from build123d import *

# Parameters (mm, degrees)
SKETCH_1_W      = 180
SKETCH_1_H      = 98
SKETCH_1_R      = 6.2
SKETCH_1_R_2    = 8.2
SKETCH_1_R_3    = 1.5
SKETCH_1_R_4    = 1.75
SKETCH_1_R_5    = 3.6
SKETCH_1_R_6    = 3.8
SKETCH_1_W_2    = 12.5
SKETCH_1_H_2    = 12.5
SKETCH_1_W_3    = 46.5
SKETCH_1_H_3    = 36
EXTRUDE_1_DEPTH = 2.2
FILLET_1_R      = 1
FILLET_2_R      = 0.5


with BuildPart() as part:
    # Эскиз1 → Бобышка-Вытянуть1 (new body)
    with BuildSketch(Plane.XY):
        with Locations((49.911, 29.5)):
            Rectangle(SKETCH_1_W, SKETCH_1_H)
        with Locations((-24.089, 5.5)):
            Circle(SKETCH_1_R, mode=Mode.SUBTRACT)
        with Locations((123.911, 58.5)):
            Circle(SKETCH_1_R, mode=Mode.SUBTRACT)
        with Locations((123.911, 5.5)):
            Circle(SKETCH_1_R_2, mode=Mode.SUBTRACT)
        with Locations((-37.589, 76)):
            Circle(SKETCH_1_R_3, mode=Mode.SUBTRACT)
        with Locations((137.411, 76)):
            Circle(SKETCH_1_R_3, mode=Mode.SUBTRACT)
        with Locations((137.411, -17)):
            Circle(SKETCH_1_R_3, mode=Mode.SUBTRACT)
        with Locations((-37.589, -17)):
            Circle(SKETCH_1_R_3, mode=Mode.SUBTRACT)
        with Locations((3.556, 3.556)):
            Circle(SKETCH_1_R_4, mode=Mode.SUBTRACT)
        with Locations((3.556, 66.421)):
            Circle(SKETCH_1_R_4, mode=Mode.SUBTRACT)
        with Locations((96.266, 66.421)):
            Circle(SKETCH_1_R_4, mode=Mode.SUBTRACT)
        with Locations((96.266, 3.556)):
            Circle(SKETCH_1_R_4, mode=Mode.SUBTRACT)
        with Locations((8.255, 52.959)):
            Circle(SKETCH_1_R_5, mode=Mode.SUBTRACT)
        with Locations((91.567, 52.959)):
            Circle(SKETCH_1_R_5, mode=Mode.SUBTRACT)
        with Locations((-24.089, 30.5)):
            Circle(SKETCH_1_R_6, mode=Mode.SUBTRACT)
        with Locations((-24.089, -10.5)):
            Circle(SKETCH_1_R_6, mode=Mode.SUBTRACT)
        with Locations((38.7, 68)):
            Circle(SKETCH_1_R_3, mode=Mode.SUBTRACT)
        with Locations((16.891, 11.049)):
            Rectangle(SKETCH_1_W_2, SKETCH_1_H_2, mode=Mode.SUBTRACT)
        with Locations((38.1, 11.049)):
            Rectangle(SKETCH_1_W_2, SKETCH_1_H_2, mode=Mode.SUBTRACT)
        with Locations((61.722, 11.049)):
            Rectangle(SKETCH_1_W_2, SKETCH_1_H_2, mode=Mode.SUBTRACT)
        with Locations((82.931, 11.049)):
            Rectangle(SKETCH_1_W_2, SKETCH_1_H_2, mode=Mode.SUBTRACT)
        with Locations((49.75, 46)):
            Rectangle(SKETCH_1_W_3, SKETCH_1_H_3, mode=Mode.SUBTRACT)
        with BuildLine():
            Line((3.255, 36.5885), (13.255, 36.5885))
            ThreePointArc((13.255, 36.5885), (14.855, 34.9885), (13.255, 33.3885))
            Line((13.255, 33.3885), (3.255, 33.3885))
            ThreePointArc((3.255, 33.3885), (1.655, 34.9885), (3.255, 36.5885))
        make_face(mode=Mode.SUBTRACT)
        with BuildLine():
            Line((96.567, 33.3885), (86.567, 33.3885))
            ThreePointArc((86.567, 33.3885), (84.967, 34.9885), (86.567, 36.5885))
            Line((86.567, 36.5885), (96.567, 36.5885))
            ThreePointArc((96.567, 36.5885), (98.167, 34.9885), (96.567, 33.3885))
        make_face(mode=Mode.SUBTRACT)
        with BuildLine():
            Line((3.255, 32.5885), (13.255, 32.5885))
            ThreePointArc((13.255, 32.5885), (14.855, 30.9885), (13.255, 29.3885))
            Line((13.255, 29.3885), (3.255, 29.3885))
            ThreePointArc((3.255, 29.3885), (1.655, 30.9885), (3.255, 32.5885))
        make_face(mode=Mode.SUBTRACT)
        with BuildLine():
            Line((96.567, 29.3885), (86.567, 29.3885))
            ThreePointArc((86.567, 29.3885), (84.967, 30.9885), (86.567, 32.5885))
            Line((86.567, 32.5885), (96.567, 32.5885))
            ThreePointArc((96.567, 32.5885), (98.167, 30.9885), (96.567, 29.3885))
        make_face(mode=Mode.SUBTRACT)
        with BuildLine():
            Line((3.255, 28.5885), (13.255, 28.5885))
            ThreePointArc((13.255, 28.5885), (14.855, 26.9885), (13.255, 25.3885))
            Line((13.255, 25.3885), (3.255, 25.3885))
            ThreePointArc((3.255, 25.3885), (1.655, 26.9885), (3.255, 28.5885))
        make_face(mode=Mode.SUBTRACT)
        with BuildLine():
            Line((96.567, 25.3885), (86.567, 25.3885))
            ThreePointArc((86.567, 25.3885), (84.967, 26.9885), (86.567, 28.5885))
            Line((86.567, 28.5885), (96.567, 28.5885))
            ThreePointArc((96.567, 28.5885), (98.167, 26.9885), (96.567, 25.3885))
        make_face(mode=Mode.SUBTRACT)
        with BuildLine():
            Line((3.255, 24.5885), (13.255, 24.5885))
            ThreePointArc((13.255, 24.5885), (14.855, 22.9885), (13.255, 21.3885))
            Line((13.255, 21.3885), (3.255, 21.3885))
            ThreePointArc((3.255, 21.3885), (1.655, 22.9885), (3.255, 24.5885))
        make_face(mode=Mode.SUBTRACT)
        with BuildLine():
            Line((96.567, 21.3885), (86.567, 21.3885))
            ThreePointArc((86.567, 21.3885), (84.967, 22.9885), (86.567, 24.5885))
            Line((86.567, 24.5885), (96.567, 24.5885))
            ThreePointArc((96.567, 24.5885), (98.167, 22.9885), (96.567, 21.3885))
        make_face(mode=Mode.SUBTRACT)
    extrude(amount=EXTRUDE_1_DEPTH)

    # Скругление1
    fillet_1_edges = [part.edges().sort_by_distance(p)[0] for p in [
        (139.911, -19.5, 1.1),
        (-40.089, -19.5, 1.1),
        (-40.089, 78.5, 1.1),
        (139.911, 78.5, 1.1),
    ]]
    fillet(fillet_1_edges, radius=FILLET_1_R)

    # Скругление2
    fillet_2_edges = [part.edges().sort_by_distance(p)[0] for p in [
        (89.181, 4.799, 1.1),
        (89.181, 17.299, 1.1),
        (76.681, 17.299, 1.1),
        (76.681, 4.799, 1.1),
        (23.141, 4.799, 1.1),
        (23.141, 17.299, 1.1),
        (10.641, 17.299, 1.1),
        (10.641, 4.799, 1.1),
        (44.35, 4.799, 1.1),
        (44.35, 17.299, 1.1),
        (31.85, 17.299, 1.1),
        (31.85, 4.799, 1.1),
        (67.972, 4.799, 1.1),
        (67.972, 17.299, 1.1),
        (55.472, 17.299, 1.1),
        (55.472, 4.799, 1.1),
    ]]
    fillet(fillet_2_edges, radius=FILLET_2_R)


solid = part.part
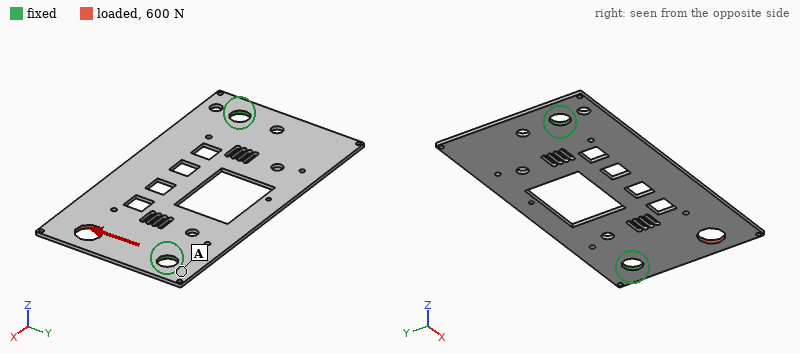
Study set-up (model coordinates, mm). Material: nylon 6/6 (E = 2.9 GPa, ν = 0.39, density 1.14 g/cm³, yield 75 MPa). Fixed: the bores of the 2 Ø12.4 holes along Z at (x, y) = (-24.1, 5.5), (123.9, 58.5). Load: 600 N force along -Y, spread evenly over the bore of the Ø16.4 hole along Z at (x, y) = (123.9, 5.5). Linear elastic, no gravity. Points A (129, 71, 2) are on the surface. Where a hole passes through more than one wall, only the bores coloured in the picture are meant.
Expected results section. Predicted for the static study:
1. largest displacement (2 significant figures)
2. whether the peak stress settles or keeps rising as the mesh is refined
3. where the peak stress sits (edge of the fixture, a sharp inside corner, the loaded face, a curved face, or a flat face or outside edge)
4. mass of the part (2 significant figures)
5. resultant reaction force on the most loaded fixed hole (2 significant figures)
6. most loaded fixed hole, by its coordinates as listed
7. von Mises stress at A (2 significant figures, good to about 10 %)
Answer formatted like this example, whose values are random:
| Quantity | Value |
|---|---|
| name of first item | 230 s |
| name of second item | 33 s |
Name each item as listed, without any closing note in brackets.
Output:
| Quantity | Value |
|---|---|
| largest displacement | 0.20 mm |
| whether the peak stress settles or keeps rising as the mesh is refined | keeps rising |
| where the peak stress sits | a sharp inside corner |
| mass of the part | 36 g |
| resultant reaction force on the most loaded fixed hole | 600 N |
| most loaded fixed hole, by its coordinates as listed | (123.9, 58.5) |
| von Mises stress at A | 2.0 MPa |
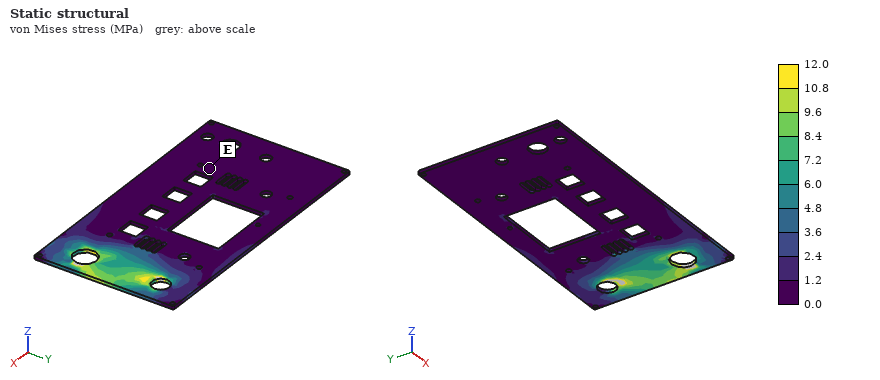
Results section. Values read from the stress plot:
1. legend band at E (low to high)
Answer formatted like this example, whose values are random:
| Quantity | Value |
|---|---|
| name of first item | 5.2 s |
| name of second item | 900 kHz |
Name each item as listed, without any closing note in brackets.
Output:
| Quantity | Value |
|---|---|
| legend band at E | 0.0 to 1.2 MPa |
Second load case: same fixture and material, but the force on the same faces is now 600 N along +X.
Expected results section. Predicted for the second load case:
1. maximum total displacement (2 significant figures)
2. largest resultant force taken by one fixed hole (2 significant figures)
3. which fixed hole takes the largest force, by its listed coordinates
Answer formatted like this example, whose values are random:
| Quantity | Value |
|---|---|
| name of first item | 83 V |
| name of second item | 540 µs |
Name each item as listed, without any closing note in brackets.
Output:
| Quantity | Value |
|---|---|
| maximum total displacement | 0.33 mm |
| largest resultant force taken by one fixed hole | 350 N |
| which fixed hole takes the largest force, by its listed coordinates | (-24.1, 5.5) |
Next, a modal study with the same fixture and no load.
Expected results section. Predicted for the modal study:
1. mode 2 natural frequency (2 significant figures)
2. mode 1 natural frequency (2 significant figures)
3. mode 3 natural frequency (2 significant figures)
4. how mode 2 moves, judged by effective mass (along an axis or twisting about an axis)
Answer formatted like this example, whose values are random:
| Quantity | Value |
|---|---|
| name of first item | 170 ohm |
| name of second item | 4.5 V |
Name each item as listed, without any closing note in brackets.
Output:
| Quantity | Value |
|---|---|
| mode 2 natural frequency | 120 Hz |
| mode 1 natural frequency | 100 Hz |
| mode 3 natural frequency | 190 Hz |
| how mode 2 moves, judged by effective mass | along Z |
